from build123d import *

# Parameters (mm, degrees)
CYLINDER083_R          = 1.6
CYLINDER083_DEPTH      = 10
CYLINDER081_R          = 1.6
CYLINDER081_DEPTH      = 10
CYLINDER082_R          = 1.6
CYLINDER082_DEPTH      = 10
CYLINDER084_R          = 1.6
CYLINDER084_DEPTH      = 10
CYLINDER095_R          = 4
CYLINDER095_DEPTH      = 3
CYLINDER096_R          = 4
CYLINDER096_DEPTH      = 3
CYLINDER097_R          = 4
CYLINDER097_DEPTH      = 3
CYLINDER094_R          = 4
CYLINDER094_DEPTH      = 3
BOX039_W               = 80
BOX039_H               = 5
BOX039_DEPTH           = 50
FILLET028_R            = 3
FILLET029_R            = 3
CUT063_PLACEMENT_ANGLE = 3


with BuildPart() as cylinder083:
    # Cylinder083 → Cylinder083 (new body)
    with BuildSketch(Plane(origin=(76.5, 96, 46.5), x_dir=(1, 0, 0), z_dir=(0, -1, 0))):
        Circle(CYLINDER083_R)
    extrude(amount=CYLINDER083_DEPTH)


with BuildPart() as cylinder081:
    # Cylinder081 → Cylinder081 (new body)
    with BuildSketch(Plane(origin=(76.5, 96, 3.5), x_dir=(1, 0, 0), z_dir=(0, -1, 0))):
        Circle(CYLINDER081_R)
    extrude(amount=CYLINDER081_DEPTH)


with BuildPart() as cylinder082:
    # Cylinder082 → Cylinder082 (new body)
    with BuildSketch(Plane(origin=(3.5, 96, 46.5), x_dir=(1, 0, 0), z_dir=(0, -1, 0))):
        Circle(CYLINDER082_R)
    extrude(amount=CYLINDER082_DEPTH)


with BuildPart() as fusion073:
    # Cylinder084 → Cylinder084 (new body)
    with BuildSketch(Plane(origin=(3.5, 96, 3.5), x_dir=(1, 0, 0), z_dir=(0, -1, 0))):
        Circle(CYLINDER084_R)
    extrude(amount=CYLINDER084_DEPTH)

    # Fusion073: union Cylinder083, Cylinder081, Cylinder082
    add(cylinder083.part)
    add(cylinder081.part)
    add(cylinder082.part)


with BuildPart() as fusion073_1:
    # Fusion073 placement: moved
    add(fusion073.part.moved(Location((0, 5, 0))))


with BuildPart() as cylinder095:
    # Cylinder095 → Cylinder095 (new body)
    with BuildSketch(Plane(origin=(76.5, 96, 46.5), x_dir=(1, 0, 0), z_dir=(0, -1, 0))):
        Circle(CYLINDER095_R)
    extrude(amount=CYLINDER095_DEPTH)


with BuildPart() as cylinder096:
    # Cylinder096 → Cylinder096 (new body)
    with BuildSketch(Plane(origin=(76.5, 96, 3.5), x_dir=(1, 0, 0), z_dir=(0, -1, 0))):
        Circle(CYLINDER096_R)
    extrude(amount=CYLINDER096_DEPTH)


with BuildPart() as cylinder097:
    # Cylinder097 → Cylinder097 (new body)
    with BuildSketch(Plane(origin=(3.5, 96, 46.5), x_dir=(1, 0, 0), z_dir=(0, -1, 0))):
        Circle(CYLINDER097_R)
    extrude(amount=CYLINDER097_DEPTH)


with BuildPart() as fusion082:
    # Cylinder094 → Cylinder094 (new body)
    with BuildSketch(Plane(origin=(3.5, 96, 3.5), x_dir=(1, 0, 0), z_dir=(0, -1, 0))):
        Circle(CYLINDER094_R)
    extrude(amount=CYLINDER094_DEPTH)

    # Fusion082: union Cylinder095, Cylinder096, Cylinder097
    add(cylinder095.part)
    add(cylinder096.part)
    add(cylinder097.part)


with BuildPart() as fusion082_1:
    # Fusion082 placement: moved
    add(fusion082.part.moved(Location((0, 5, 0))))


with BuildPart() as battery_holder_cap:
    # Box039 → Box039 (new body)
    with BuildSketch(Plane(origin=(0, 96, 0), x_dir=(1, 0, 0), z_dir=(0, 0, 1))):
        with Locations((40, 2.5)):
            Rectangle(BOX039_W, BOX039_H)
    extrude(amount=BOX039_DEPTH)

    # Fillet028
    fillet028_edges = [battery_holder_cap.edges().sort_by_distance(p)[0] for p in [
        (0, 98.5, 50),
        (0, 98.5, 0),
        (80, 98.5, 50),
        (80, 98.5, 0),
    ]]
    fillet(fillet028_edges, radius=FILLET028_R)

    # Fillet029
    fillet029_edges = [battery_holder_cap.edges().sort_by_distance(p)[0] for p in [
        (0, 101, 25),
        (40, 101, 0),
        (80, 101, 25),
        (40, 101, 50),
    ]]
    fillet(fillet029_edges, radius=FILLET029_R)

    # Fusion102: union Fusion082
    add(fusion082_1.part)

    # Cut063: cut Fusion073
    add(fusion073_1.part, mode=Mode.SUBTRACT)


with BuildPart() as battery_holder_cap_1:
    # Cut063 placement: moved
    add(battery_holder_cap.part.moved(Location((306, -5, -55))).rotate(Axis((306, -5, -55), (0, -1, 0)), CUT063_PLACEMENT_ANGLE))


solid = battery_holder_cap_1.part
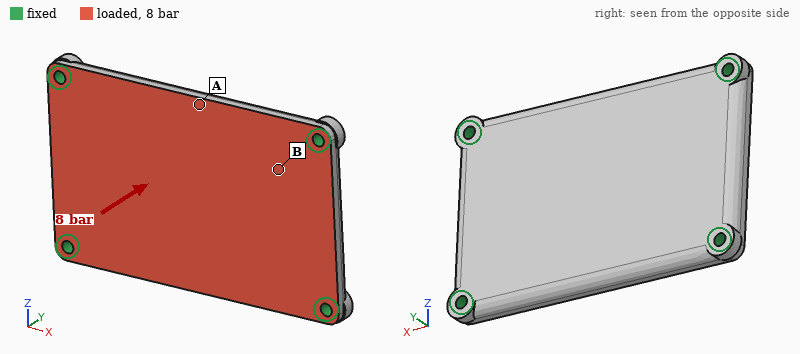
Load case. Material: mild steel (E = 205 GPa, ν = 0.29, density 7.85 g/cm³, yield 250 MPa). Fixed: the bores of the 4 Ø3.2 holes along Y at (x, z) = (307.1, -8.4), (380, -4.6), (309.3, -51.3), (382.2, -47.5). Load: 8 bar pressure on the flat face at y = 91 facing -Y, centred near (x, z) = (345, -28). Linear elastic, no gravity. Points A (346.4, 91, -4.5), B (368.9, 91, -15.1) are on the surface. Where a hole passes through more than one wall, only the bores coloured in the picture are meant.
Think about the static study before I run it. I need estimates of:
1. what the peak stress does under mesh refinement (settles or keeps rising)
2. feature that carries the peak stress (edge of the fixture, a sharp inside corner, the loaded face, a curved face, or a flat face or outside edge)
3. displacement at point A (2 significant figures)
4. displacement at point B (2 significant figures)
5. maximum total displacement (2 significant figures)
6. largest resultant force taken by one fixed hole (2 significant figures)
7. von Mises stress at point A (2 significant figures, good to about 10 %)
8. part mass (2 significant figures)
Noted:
keeps rising
edge of the fixture
45 µm
21 µm
47 µm
790 N
59 MPa
150 g
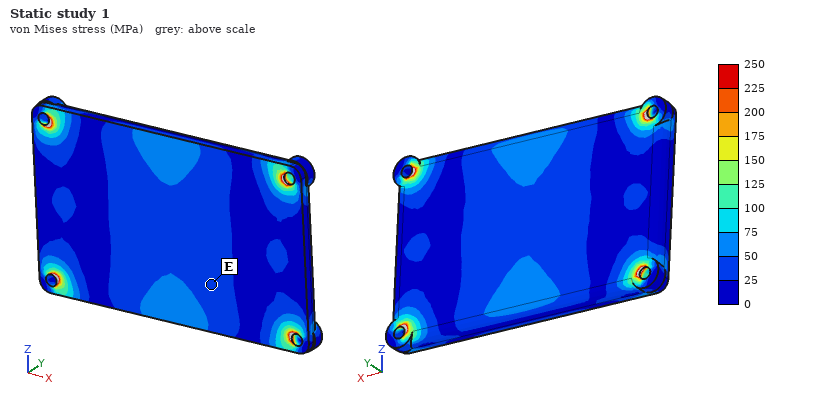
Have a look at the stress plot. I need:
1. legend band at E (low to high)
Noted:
25 to 50 MPa
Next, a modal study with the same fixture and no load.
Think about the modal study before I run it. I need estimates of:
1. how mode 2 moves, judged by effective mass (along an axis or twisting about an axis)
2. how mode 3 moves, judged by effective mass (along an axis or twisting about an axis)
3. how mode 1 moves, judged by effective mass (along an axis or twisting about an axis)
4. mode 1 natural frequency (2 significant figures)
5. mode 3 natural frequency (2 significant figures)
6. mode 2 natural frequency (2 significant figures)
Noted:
twisting about X
twisting about Z
along Y
3800 Hz
9800 Hz
6500 Hz
